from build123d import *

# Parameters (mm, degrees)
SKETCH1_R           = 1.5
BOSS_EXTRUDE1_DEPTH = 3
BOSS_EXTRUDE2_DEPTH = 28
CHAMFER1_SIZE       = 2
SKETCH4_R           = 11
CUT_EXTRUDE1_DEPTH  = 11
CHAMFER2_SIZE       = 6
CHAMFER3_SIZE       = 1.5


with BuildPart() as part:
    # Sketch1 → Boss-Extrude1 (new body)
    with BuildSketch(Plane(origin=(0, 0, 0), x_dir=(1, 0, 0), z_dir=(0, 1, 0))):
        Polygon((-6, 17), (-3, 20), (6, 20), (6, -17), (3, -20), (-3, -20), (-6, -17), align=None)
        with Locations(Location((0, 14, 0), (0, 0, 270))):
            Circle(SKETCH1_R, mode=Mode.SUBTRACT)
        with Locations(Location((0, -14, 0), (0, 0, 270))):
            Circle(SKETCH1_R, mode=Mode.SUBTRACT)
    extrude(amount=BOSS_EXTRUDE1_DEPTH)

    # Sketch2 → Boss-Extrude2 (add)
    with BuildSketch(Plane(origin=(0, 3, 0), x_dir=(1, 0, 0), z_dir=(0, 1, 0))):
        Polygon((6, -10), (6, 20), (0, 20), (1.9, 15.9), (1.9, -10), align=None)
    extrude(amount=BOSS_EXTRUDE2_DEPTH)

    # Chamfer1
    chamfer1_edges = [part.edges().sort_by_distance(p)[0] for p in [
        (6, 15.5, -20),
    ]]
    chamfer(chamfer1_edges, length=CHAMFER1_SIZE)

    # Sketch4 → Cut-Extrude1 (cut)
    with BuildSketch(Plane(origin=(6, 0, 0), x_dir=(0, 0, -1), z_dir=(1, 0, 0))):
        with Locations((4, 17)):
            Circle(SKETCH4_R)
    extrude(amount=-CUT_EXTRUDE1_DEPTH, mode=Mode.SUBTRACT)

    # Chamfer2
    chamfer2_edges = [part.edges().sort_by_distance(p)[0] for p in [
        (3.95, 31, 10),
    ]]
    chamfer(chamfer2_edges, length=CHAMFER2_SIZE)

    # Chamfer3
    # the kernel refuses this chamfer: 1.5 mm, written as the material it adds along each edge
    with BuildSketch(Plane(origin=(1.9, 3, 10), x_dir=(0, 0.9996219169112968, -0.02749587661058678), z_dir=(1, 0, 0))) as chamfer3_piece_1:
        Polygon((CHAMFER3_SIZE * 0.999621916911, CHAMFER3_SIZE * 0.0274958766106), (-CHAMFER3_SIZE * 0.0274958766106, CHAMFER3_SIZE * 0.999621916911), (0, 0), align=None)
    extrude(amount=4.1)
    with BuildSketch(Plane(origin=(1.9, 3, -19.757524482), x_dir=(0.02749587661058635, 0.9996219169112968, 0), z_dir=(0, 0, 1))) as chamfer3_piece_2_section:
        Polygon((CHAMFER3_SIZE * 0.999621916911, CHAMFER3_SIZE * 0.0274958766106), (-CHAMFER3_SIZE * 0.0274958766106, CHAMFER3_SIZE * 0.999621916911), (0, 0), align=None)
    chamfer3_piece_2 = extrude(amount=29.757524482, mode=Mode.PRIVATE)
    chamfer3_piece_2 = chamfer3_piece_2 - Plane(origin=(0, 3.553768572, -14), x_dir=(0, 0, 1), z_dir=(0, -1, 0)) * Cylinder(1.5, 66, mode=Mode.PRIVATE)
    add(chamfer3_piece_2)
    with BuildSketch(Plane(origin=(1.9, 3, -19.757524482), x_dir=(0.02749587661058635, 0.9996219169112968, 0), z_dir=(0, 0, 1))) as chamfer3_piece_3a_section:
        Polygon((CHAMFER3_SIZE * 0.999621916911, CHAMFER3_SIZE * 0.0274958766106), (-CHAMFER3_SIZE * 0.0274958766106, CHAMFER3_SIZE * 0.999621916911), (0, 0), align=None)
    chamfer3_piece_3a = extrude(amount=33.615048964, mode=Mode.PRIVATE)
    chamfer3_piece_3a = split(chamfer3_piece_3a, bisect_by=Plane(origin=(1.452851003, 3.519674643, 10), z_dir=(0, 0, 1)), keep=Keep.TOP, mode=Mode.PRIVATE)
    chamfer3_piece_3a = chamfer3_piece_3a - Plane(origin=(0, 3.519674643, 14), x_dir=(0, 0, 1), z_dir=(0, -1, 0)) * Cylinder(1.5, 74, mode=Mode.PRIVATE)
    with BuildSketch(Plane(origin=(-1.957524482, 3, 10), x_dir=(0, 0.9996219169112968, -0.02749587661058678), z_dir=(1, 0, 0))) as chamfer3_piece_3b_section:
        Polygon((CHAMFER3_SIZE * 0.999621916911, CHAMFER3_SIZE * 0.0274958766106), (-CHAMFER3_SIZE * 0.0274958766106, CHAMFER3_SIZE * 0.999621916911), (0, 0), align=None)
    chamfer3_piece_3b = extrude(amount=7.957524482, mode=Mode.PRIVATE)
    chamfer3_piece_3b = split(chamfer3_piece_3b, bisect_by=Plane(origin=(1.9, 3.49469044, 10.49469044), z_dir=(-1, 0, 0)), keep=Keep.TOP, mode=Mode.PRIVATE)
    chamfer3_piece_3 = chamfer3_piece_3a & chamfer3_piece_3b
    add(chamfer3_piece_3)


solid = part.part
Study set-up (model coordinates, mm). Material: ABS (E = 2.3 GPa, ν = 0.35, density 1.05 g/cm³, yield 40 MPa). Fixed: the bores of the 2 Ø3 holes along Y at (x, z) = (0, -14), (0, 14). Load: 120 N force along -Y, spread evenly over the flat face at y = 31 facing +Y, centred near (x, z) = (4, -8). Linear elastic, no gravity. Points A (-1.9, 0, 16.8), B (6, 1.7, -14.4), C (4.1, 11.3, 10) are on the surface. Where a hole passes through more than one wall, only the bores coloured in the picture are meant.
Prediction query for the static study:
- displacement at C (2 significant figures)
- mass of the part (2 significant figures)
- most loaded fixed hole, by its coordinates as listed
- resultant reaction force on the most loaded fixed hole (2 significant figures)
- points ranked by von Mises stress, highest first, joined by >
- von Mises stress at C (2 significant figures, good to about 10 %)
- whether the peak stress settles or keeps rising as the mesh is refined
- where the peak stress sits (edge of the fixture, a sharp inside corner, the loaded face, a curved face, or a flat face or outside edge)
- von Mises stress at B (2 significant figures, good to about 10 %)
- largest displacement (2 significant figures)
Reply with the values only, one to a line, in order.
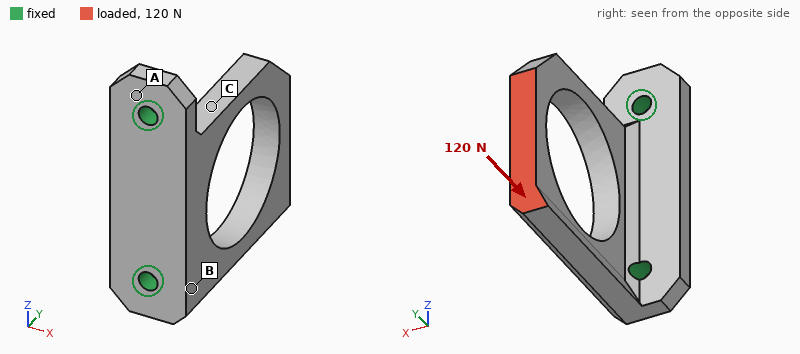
0.084 mm
3.4 g
(0, -14)
85 N
C > B > A
7.1 MPa
keeps rising
edge of the fixture
2.5 MPa
0.27 mm
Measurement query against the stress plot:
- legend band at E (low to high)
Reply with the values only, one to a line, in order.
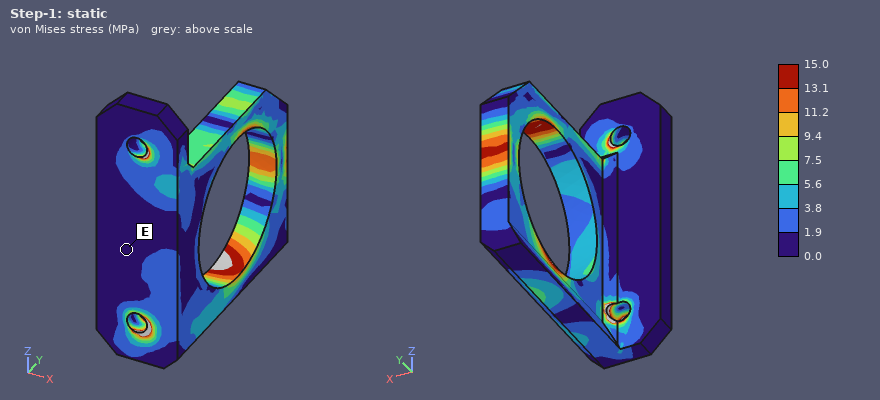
0.0 to 1.9 MPa
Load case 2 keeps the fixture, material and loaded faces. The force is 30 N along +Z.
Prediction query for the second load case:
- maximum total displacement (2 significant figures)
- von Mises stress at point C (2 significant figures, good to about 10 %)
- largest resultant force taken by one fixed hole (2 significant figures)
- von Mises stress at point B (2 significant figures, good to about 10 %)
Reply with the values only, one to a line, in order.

0.25 mm
7.6 MPa
33 N
2.1 MPa
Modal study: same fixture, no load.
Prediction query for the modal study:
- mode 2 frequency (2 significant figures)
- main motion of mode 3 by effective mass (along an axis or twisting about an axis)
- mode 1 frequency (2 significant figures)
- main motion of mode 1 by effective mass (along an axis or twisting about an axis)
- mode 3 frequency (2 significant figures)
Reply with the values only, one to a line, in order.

1900 Hz
along Z
910 Hz
along X
2300 Hz
